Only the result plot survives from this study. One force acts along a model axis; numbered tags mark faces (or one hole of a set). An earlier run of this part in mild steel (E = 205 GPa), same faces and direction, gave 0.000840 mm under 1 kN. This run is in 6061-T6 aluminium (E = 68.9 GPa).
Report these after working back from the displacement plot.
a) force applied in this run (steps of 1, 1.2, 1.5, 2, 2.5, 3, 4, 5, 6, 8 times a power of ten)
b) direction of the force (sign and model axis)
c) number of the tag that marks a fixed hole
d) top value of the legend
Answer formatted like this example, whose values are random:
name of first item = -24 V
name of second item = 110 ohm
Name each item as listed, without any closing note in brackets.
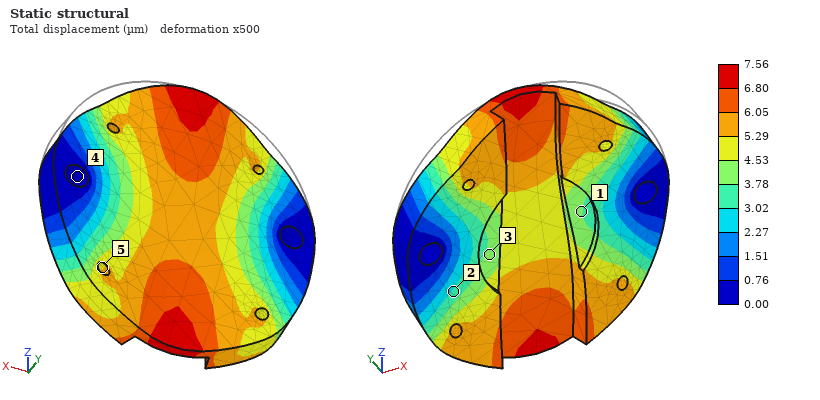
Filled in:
force applied in this run = 3 kN
direction of the force = -Z
number of the tag that marks a fixed hole = 4
top value of the legend = 7.56 µm
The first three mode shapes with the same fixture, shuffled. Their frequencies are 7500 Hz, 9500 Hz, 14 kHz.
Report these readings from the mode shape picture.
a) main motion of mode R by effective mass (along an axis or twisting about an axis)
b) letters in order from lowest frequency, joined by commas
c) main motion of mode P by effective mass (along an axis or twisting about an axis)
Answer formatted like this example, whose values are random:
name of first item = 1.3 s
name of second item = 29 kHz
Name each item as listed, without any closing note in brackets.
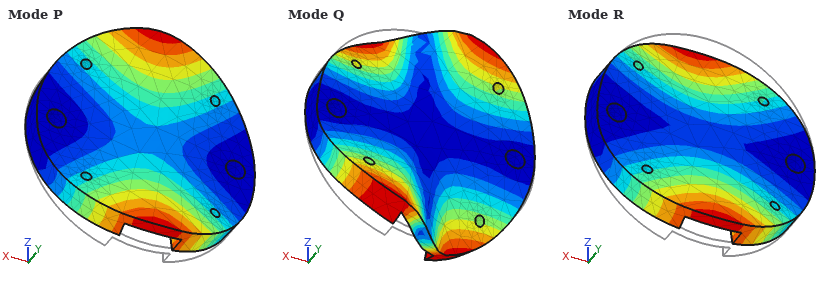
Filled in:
main motion of mode R by effective mass = twisting about X
letters in order from lowest frequency, joined by commas = R, P, Q
main motion of mode P by effective mass = along Y
